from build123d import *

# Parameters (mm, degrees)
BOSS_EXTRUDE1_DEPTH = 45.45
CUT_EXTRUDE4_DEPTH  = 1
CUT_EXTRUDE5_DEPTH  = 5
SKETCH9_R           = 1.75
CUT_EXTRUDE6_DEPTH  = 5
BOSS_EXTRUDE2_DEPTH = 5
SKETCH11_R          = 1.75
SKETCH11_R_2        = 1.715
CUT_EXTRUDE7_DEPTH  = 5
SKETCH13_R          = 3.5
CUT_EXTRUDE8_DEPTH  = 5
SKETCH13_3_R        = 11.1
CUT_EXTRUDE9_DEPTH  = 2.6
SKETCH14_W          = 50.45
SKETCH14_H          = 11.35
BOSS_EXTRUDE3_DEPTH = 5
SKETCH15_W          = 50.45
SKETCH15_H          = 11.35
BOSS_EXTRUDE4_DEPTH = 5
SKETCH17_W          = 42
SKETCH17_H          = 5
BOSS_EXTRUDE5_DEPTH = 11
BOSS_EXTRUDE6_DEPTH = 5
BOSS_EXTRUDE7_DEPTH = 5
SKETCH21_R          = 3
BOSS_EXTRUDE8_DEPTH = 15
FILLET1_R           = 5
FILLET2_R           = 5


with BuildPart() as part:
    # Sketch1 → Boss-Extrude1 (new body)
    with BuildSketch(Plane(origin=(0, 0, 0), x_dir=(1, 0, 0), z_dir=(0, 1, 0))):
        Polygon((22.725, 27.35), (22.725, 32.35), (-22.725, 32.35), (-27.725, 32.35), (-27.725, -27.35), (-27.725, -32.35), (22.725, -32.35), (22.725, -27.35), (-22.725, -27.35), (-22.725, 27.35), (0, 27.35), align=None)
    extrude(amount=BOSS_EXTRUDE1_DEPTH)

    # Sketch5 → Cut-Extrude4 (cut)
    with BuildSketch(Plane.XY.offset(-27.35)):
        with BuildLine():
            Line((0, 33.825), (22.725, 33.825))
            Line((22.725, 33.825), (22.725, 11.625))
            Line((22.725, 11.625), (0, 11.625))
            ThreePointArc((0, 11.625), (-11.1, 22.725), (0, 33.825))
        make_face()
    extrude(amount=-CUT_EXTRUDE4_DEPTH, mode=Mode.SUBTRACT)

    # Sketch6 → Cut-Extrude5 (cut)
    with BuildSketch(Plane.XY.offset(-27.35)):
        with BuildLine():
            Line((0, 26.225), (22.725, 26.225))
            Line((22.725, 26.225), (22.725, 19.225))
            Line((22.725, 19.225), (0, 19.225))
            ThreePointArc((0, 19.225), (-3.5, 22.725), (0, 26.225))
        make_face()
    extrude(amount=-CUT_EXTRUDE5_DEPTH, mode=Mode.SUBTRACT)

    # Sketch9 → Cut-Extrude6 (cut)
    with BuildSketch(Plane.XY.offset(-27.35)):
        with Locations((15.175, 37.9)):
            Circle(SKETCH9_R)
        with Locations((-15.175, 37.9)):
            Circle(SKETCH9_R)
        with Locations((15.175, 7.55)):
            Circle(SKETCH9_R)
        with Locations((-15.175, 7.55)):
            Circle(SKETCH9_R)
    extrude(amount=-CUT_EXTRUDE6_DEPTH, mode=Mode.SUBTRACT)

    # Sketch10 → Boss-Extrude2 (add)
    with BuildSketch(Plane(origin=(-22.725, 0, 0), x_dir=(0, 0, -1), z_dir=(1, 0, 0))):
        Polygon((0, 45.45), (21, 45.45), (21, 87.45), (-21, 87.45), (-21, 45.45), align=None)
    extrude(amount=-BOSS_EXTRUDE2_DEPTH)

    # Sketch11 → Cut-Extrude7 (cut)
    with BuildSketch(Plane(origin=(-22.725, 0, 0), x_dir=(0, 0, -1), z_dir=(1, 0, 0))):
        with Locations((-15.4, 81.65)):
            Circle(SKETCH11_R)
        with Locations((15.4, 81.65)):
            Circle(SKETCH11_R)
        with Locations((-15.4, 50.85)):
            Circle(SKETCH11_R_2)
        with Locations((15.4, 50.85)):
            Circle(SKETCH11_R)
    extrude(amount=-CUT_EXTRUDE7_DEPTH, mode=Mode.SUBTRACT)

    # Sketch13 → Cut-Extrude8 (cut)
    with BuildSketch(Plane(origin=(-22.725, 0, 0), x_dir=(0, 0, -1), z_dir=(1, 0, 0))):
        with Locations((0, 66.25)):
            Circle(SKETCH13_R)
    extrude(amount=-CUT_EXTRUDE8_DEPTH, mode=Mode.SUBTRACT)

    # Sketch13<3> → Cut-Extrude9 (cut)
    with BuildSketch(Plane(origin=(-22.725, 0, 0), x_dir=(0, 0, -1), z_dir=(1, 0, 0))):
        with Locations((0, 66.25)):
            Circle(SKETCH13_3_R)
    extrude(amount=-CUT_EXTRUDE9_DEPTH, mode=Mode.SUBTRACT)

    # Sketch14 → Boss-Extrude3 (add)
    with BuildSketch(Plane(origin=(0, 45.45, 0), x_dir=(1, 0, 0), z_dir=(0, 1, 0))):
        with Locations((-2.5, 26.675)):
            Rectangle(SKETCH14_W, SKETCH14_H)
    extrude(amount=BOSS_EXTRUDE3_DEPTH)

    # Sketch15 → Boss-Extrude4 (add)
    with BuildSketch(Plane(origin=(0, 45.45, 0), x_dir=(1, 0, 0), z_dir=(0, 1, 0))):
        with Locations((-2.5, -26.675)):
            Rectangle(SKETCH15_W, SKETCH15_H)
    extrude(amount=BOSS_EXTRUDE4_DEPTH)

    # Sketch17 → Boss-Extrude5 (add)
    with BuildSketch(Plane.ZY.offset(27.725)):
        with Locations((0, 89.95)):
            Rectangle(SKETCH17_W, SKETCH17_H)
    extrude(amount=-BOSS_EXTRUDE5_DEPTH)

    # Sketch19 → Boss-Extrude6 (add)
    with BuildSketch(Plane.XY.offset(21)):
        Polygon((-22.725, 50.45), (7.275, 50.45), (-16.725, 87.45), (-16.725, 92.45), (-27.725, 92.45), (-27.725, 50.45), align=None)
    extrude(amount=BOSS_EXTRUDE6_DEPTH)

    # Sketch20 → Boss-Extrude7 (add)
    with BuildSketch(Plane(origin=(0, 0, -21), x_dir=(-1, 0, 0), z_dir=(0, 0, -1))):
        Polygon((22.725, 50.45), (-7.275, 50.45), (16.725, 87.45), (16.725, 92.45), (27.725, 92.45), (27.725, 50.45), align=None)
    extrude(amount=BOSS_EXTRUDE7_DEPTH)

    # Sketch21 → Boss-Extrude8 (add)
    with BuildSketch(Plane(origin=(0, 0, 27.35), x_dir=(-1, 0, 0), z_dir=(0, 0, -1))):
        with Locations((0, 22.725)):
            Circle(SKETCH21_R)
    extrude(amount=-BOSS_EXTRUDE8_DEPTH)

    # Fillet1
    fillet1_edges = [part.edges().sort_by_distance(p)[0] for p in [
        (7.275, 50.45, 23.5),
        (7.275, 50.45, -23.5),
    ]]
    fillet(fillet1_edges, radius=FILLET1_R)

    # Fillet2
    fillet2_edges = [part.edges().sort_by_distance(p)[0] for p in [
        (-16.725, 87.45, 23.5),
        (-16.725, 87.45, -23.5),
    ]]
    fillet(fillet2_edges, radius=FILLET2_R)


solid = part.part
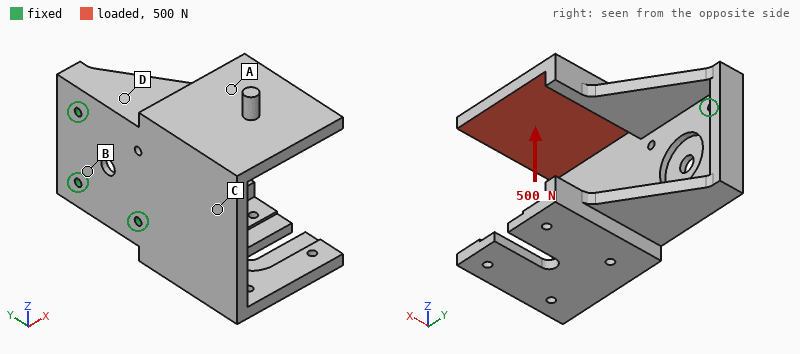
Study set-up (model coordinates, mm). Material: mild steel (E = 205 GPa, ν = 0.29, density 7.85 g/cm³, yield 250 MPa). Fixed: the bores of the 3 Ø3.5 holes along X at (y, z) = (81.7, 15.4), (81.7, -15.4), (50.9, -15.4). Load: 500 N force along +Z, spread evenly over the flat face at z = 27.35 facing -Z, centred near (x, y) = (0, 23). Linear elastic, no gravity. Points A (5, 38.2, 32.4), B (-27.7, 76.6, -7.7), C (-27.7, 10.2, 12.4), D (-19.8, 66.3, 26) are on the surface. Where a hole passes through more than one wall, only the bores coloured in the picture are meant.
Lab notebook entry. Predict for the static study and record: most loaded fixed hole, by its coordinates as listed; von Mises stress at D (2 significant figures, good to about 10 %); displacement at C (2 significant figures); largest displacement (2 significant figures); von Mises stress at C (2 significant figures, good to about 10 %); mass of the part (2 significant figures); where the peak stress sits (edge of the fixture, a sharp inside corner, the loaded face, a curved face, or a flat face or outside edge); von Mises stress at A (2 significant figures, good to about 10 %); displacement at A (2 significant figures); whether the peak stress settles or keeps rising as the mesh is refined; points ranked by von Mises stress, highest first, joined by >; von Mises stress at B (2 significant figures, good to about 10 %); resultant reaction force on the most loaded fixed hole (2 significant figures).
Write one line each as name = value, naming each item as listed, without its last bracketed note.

most loaded fixed hole, by its coordinates as listed = (50.9, -15.4)
von Mises stress at D = 38 MPa
displacement at C = 0.028 mm
largest displacement = 0.17 mm
von Mises stress at C = 24 MPa
mass of the part = 460 g
where the peak stress sits = edge of the fixture
von Mises stress at A = 16 MPa
displacement at A = 0.092 mm
whether the peak stress settles or keeps rising as the mesh is refined = keeps rising
points ranked by von Mises stress, highest first, joined by > = D > C > A > B
von Mises stress at B = 6.1 MPa
resultant reaction force on the most loaded fixed hole = 760 N
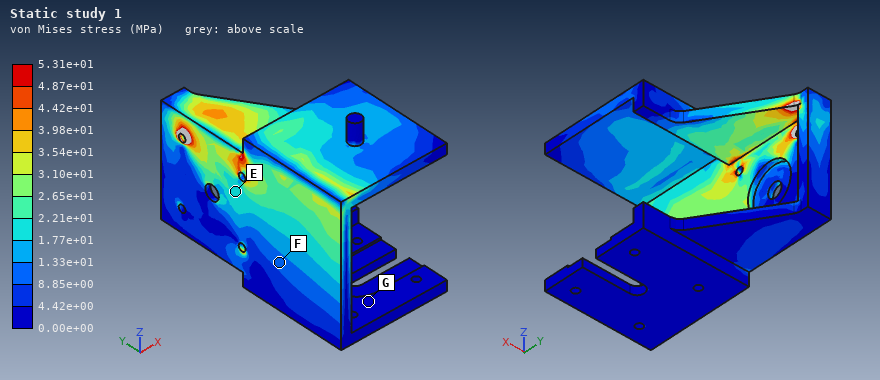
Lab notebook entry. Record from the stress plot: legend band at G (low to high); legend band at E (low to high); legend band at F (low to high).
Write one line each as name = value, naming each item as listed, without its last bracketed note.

legend band at G = 0.00e+00 to 4.42e+00 MPa
legend band at E = 1.77e+01 to 2.21e+01 MPa
legend band at F = 8.85e+00 to 1.33e+01 MPa
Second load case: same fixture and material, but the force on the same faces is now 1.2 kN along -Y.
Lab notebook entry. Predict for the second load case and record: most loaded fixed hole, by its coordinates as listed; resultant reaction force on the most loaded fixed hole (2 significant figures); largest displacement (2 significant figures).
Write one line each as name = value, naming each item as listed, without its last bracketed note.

most loaded fixed hole, by its coordinates as listed = (81.7, 15.4)
resultant reaction force on the most loaded fixed hole = 1.5 kN
largest displacement = 0.17 mm
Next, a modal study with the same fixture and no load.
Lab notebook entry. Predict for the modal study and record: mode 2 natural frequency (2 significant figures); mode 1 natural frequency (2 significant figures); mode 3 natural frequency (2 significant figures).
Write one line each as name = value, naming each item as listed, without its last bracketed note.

mode 2 natural frequency = 1400 Hz
mode 1 natural frequency = 760 Hz
mode 3 natural frequency = 1600 Hz
